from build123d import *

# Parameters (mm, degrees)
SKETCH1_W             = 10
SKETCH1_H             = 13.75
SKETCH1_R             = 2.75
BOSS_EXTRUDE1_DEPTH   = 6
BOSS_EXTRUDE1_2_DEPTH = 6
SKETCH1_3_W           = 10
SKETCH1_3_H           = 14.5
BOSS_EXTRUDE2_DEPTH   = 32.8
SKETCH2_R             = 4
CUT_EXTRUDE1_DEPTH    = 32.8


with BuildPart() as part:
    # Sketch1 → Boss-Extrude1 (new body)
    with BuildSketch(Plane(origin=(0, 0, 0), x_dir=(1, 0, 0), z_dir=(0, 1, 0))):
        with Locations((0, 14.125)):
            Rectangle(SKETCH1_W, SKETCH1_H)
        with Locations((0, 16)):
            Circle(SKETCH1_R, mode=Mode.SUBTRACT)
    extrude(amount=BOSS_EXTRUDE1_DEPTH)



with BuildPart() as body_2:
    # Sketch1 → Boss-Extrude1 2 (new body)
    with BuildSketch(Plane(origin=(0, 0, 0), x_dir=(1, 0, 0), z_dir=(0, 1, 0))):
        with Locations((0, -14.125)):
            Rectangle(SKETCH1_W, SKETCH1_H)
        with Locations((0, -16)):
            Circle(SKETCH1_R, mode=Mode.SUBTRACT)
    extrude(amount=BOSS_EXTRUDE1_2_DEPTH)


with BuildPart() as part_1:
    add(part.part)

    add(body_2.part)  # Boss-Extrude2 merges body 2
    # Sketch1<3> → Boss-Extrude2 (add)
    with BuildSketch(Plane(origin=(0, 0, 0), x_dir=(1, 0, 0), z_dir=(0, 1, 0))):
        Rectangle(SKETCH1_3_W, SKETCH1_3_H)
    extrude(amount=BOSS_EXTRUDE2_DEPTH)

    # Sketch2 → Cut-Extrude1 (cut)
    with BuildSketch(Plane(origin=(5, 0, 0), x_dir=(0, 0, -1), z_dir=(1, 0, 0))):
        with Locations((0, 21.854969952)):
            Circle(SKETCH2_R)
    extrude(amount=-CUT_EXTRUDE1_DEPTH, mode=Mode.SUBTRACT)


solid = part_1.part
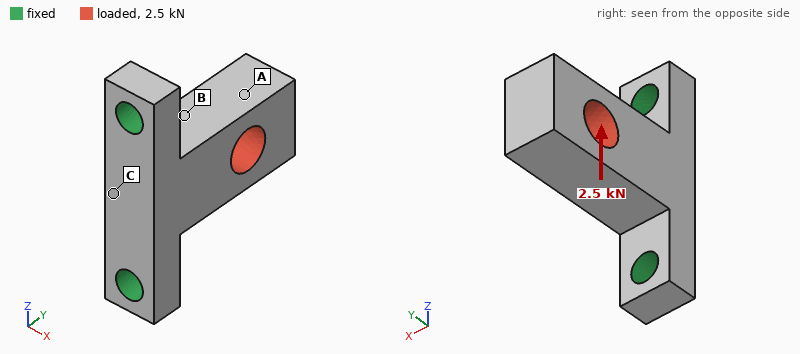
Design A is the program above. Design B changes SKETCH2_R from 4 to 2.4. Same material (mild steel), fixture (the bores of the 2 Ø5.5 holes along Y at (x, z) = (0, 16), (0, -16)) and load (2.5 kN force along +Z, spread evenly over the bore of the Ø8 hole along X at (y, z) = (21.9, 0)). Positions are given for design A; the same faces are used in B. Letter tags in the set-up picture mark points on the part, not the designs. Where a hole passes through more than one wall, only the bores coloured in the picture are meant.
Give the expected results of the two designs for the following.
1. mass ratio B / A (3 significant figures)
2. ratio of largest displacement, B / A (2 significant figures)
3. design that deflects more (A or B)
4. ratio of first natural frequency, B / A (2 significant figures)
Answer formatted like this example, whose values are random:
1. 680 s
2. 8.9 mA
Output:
1. 1.06
2. 0.91
3. A
4. 0.96
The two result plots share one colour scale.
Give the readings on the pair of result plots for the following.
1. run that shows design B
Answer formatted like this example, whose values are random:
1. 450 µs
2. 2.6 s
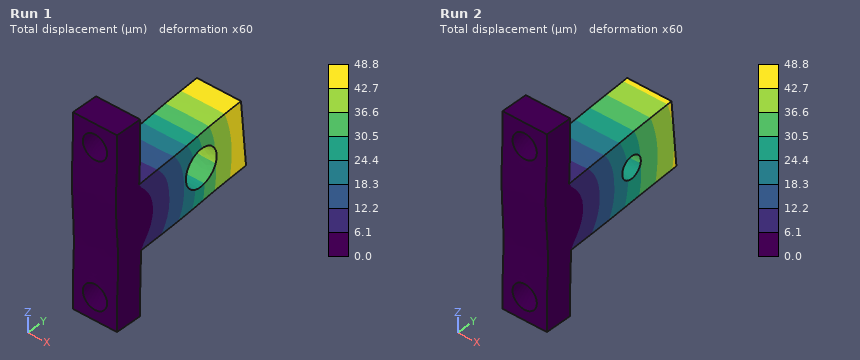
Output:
1. Run 2
